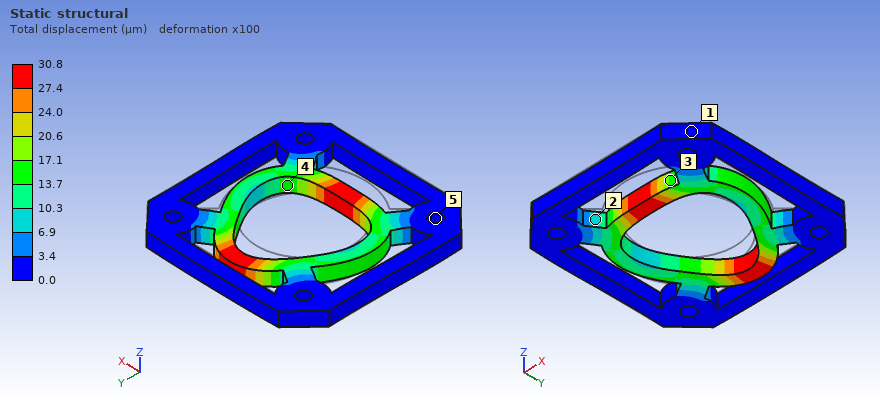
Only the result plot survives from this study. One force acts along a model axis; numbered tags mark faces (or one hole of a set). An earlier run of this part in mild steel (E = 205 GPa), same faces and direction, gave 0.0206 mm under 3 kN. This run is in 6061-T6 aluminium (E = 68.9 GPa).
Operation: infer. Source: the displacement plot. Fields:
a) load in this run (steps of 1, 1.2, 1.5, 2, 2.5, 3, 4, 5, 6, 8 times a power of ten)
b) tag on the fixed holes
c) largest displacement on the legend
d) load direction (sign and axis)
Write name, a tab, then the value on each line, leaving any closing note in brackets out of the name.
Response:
load in this run	1.5 kN
tag on the fixed holes	5
largest displacement on the legend	30.8 µm
load direction	+Y
